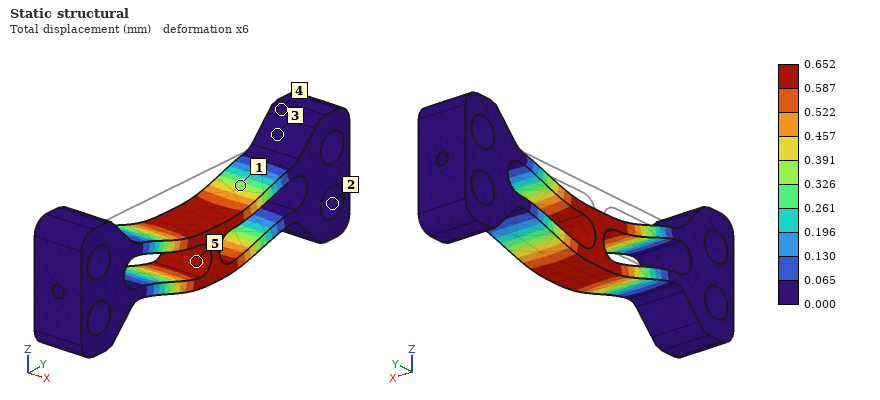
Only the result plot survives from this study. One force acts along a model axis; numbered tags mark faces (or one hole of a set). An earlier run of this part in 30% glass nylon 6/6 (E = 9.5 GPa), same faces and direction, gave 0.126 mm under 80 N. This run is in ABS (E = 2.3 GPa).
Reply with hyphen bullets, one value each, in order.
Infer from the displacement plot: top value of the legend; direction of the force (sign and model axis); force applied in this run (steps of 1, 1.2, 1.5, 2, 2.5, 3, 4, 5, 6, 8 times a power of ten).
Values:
- 0.652 mm
- -Z
- 100 N
